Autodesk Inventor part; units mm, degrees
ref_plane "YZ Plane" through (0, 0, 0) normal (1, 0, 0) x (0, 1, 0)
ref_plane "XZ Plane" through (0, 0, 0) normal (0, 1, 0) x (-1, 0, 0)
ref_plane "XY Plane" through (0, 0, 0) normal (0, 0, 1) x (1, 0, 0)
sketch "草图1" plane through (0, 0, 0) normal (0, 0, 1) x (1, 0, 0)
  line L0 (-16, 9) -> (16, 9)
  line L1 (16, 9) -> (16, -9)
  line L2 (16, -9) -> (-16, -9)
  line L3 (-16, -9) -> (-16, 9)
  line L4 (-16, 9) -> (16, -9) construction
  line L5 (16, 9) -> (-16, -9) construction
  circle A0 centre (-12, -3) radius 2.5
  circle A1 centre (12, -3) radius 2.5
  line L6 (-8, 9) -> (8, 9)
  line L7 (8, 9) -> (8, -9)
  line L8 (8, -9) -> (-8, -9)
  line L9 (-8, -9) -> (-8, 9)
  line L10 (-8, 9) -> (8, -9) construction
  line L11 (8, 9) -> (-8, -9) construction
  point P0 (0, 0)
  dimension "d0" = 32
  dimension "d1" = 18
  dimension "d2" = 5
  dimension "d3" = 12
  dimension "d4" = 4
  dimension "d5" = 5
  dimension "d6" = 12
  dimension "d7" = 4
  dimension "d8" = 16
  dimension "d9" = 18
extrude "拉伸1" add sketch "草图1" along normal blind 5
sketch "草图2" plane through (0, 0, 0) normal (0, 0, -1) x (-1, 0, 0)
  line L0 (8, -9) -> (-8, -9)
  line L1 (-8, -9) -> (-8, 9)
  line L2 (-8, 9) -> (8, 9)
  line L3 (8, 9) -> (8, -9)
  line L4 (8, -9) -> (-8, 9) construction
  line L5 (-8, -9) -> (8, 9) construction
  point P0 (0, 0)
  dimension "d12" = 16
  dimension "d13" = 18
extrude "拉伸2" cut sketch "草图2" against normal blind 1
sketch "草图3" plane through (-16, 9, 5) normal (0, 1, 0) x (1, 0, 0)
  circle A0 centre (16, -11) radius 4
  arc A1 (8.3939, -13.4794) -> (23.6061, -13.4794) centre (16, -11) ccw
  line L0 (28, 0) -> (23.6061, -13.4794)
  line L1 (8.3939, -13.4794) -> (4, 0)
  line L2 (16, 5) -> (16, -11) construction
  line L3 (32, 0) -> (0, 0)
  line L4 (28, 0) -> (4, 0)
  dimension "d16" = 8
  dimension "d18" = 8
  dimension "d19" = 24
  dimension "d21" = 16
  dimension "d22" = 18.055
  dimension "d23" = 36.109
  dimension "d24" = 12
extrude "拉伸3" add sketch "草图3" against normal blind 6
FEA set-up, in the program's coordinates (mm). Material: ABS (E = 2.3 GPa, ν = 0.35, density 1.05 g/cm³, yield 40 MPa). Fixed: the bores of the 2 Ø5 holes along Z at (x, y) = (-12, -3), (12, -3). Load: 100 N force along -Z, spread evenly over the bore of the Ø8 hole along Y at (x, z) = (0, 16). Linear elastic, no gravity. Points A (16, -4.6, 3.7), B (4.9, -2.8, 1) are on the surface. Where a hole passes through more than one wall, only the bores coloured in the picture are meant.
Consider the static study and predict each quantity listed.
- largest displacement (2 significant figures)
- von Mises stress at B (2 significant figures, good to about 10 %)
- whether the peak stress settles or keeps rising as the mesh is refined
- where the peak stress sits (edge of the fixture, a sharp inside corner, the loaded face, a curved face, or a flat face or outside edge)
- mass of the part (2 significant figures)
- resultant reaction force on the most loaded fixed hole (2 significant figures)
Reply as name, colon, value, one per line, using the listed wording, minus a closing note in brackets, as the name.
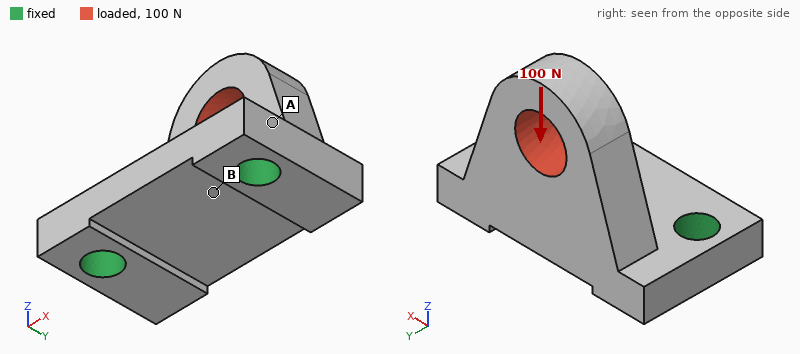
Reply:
largest displacement: 0.14 mm
von Mises stress at B: 1.8 MPa
whether the peak stress settles or keeps rising as the mesh is refined: keeps rising
where the peak stress sits: edge of the fixture
mass of the part: 4.3 g
resultant reaction force on the most loaded fixed hole: 51 N
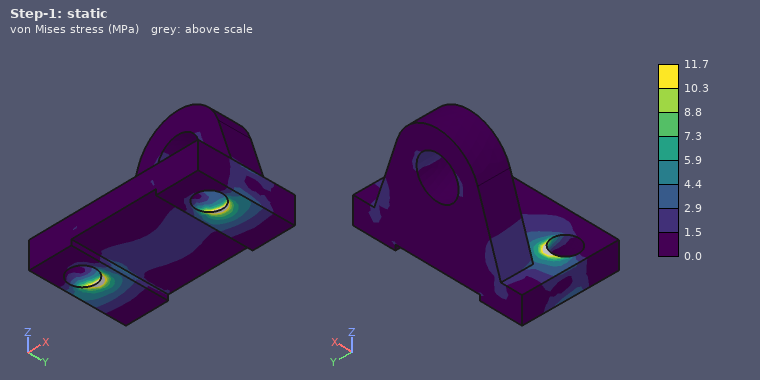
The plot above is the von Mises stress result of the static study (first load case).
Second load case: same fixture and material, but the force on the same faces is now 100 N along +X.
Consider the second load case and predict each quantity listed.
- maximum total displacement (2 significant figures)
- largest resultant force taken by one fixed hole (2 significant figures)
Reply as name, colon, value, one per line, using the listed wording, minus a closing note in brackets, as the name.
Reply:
maximum total displacement: 89 µm
largest resultant force taken by one fixed hole: 82 N
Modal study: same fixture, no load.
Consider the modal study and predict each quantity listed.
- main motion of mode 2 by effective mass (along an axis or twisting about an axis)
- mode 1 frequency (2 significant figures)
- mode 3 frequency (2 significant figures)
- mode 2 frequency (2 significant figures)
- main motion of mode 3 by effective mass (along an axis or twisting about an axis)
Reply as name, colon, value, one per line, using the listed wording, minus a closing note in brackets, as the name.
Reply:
main motion of mode 2 by effective mass: along X
mode 1 frequency: 2400 Hz
mode 3 frequency: 6600 Hz
mode 2 frequency: 5400 Hz
main motion of mode 3 by effective mass: along Z
